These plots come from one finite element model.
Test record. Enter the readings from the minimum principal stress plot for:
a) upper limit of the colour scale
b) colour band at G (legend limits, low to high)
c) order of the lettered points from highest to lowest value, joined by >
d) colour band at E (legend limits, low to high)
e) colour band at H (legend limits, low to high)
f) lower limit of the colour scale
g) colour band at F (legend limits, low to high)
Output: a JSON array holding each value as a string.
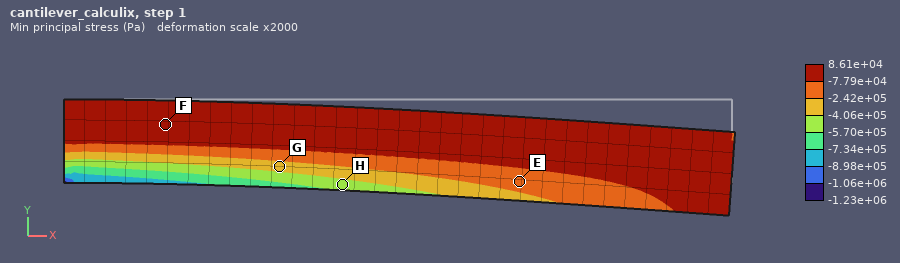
["8.61e+04 Pa", "-4.06e+05 to -2.42e+05 Pa", "F > E > G > H", "-2.42e+05 to -7.79e+04 Pa", "-5.70e+05 to -4.06e+05 Pa", "-1.23e+06 Pa", "-7.79e+04 to 8.61e+04 Pa"]
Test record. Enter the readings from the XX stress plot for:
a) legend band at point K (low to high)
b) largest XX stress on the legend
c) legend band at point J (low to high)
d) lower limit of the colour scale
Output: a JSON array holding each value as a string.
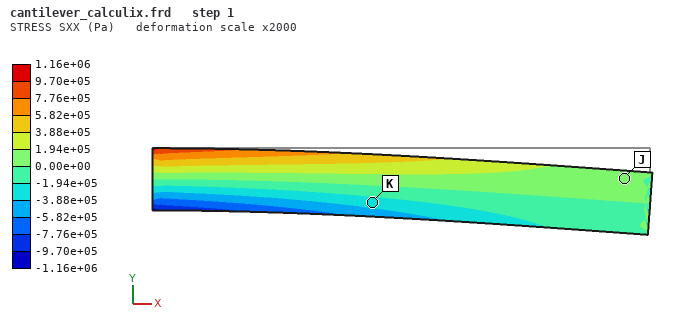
["-3.88e+05 to -1.94e+05 Pa", "1.16e+06 Pa", "0.00e+00 to 1.94e+05 Pa", "-1.16e+06 Pa"]
